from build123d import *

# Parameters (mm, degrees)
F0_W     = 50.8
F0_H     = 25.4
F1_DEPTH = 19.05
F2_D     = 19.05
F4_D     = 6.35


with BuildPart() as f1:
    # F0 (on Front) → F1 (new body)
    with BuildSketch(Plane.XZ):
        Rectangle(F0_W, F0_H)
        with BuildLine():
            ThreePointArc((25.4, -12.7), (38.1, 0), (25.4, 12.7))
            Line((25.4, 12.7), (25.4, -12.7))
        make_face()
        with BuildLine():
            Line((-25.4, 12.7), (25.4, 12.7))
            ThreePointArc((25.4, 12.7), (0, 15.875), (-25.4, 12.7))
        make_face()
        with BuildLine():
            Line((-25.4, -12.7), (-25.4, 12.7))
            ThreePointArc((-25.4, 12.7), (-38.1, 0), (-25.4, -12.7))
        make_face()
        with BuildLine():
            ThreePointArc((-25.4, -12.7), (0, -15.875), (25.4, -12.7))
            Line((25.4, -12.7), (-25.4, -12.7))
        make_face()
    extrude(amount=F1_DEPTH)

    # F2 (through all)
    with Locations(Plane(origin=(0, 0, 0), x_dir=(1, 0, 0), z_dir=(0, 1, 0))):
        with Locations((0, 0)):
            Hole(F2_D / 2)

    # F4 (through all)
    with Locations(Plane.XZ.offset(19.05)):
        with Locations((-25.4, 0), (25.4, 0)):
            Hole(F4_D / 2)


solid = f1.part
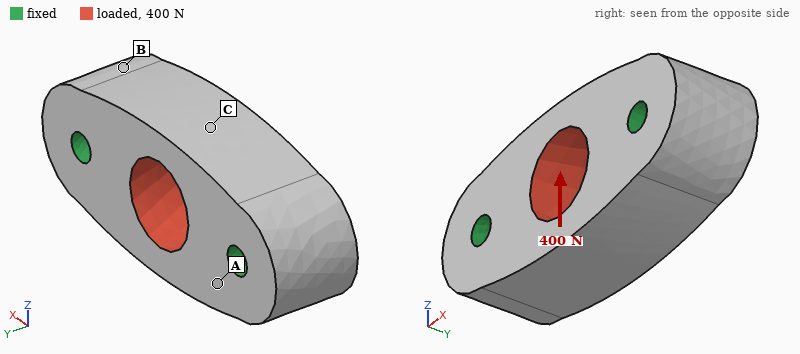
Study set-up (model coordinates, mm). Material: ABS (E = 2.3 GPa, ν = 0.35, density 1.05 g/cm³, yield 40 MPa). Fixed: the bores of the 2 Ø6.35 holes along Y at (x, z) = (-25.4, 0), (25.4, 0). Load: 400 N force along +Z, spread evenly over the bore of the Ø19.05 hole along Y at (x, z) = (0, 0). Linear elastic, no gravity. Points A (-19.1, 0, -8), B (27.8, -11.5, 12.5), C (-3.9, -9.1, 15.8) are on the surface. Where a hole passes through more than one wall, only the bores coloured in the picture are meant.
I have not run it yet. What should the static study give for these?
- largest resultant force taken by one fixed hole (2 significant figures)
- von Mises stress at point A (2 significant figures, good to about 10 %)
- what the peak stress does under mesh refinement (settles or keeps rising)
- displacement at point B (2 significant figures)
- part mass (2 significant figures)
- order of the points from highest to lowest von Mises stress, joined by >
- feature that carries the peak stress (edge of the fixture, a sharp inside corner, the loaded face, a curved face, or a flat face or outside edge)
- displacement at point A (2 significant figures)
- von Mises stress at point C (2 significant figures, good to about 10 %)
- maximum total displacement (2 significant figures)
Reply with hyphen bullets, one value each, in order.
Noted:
- 200 N
- 0.65 MPa
- keeps rising
- 4.3 µm
- 33 g
- C > A > B
- edge of the fixture
- 5.2 µm
- 1.3 MPa
- 18 µm
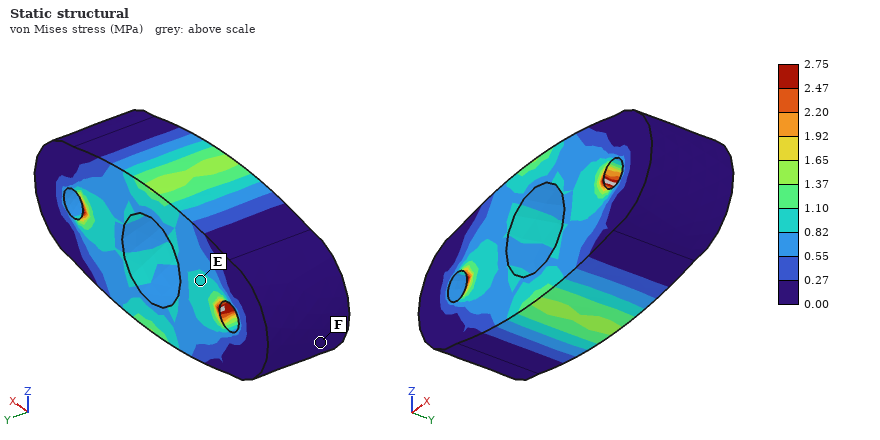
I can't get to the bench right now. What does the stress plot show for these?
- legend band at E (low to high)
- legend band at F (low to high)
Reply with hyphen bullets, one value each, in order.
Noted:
- 0.82 to 1.10 MPa
- 0.00 to 0.27 MPa
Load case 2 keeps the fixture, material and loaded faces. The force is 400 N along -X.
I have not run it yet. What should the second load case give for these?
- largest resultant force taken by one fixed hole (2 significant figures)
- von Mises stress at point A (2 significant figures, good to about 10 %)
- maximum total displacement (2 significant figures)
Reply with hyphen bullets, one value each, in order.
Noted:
- 200 N
- 0.31 MPa
- 5.5 µm
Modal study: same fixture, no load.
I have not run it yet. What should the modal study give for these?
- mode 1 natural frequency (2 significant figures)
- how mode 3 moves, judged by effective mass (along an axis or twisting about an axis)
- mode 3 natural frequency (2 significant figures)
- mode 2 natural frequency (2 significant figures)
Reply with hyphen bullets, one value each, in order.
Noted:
- 6500 Hz
- along Z
- 7400 Hz
- 6700 Hz
